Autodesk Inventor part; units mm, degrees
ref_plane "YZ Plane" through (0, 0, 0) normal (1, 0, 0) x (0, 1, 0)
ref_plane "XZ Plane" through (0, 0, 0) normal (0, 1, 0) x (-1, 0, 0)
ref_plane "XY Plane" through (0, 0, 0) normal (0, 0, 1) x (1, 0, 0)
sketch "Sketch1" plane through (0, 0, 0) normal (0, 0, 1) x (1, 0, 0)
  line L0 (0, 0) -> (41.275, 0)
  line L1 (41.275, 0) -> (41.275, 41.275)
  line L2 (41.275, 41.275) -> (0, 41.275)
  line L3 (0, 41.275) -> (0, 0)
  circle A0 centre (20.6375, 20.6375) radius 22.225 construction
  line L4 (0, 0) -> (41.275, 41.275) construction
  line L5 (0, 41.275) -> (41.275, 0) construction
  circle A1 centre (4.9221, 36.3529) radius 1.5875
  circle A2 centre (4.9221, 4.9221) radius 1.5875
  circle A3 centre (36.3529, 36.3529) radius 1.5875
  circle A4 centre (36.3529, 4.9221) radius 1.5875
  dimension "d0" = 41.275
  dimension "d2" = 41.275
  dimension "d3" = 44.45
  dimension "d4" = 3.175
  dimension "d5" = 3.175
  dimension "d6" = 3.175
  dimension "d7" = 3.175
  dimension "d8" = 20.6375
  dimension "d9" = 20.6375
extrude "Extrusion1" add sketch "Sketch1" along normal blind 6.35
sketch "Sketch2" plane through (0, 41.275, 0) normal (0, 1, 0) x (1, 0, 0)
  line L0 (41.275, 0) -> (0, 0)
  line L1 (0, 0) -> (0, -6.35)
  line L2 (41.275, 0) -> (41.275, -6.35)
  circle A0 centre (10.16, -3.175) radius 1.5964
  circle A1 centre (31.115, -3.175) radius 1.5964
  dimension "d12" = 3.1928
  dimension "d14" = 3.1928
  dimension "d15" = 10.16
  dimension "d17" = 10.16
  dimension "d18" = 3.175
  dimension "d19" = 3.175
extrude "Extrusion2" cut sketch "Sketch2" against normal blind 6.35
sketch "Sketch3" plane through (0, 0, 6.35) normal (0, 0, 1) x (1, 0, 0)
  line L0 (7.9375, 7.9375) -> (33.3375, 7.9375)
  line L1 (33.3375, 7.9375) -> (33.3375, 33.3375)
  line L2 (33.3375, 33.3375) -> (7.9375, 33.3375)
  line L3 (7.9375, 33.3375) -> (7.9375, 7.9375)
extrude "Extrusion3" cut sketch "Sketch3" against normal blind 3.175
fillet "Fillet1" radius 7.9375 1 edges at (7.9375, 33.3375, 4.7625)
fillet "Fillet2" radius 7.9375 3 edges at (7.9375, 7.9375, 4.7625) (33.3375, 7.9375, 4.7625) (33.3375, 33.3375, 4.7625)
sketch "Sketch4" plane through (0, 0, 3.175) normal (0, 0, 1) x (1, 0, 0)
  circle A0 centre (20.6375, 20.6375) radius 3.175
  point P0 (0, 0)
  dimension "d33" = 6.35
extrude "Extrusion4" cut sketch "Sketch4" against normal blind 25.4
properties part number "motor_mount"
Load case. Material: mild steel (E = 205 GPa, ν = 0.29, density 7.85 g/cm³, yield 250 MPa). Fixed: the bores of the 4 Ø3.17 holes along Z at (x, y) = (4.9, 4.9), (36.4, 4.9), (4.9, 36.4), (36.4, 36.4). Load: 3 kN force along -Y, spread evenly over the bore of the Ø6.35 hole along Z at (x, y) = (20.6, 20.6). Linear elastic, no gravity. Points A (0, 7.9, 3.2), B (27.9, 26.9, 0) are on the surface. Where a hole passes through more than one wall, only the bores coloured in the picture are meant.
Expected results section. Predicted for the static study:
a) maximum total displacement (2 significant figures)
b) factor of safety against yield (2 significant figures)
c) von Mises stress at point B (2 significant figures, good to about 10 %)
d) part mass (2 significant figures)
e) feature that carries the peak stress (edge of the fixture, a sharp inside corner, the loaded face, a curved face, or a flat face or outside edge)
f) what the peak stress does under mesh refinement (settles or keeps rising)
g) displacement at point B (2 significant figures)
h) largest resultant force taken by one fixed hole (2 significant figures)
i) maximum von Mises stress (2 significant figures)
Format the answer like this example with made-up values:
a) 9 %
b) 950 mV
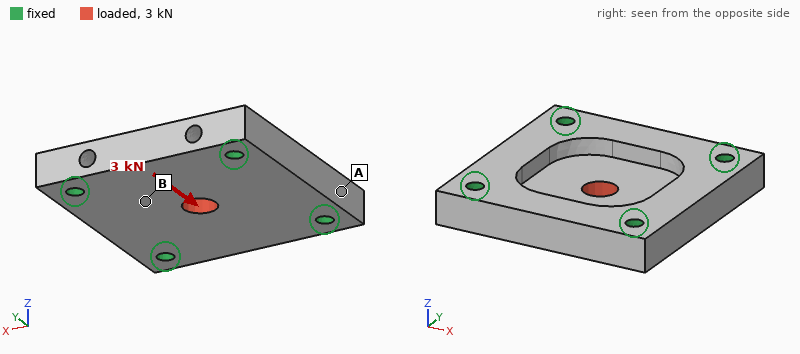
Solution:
a) 3.1 µm
b) 3.0
c) 23 MPa
d) 67 g
e) the loaded face
f) settles
g) 1.4 µm
h) 830 N
i) 83 MPa
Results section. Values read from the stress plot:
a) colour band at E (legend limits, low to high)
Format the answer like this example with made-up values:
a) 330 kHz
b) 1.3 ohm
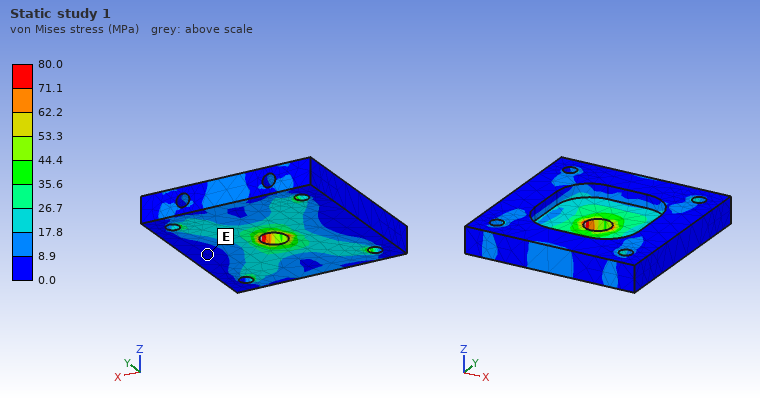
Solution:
a) 0.0 to 8.9 MPa
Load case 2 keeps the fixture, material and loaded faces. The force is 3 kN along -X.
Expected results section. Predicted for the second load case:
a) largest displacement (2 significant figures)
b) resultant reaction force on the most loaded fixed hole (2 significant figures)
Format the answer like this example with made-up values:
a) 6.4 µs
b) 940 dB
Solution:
a) 3.1 µm
b) 840 N
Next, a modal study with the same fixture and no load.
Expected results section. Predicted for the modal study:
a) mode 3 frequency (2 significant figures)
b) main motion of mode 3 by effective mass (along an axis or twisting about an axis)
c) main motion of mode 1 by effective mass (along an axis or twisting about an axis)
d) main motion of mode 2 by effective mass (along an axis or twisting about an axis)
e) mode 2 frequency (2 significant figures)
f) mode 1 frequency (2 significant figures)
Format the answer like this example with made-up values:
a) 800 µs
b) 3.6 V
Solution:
a) 28 kHz
b) twisting about Y
c) along Z
d) twisting about X
e) 26 kHz
f) 20 kHz
